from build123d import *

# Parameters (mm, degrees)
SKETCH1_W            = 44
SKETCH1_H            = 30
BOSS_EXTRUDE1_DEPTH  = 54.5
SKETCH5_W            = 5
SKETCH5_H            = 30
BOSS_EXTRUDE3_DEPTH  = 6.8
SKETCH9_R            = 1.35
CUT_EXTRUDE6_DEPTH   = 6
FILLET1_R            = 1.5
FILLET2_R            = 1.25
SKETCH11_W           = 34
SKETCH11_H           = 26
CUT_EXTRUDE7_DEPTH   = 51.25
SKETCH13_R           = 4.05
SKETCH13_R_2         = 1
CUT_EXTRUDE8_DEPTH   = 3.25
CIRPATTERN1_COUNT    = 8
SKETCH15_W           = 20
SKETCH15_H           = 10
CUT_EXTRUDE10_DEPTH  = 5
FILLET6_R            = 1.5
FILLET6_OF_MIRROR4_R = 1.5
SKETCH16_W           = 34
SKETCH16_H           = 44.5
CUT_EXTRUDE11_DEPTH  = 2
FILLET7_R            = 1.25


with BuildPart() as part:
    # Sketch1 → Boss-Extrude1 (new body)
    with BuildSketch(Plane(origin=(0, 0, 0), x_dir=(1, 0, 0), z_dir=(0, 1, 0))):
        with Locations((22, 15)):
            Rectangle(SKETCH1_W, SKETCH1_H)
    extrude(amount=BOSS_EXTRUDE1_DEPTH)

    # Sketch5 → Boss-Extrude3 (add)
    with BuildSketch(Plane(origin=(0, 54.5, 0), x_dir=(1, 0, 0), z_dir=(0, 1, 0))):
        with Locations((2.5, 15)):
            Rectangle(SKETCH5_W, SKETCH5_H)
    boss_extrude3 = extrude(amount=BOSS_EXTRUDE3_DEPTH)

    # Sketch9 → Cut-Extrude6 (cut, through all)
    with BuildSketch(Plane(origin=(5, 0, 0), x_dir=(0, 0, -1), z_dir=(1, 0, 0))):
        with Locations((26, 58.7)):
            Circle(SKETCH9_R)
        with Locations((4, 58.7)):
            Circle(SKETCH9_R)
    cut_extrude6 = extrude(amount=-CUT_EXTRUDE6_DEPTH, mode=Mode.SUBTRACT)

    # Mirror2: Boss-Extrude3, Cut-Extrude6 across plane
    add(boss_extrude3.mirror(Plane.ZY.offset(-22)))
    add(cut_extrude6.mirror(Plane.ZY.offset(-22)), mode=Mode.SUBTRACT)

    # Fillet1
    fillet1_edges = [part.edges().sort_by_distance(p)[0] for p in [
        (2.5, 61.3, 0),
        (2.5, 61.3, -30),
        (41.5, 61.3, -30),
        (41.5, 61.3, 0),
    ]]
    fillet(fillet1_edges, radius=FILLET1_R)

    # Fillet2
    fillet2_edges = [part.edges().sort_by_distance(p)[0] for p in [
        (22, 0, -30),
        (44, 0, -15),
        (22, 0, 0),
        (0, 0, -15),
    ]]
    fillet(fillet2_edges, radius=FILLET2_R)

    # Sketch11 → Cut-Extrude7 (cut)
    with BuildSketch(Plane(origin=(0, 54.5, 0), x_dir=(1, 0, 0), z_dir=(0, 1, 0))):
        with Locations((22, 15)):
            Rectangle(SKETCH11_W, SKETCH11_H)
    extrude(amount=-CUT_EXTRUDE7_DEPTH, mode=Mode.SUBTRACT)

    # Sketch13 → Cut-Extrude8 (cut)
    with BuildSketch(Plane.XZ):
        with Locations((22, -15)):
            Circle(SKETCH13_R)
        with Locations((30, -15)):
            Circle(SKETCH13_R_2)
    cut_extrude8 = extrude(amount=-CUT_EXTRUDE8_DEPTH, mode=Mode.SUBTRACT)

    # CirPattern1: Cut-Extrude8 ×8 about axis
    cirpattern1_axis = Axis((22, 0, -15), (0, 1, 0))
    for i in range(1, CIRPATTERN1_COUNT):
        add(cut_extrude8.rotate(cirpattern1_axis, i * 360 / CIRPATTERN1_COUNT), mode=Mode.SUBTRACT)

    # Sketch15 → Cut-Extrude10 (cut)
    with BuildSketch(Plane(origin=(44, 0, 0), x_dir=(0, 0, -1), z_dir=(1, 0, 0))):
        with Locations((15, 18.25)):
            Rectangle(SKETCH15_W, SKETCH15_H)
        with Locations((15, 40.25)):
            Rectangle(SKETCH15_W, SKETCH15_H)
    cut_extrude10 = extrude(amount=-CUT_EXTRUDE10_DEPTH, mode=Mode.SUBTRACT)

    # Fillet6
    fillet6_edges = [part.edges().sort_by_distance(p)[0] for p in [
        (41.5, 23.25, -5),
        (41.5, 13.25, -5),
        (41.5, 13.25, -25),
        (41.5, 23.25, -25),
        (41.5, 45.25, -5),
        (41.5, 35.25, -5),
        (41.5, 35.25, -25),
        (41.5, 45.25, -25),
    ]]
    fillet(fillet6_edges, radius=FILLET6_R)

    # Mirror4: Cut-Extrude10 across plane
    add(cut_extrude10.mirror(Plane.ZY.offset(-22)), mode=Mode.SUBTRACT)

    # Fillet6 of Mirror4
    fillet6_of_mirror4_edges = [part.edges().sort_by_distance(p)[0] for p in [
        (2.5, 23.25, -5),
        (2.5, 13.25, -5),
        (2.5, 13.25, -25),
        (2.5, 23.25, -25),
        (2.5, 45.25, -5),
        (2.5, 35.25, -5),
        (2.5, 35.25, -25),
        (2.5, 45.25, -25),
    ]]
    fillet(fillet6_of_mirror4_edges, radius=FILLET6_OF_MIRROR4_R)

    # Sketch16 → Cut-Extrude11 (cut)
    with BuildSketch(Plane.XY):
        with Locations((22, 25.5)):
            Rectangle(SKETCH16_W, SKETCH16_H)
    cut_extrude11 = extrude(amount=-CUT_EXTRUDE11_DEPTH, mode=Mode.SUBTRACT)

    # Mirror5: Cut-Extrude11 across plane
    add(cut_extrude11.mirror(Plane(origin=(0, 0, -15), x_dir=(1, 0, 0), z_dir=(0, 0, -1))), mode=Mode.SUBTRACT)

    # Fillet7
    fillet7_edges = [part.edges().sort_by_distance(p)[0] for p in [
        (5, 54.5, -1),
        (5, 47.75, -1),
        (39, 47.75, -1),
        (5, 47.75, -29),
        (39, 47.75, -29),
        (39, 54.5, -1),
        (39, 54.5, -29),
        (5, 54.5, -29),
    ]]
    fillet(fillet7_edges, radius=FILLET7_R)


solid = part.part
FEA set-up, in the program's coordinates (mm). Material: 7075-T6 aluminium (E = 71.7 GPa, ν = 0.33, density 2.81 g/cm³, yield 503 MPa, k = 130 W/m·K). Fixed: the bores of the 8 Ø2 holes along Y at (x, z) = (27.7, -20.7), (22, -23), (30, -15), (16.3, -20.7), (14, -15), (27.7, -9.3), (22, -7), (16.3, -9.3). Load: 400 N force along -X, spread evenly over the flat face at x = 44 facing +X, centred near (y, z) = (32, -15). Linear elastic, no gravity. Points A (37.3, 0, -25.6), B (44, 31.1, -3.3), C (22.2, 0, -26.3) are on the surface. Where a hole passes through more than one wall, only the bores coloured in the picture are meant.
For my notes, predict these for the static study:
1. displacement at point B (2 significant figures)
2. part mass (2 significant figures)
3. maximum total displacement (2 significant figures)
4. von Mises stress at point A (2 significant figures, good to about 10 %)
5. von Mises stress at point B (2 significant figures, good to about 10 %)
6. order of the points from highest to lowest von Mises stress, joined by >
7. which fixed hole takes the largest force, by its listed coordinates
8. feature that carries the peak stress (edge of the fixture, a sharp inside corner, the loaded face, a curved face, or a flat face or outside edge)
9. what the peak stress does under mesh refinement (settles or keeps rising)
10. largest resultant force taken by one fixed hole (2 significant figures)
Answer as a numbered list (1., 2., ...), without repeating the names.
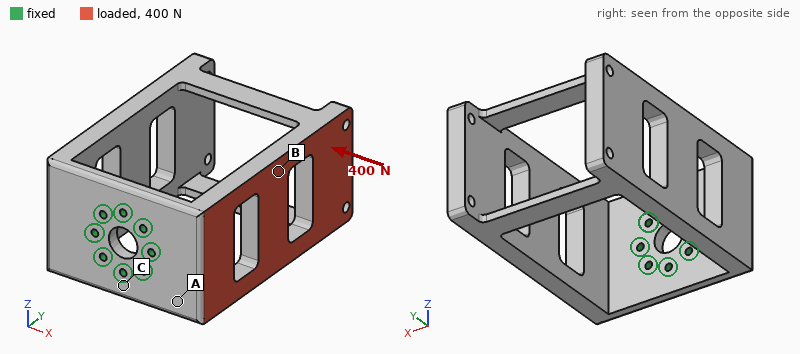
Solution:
1. 0.30 mm
2. 51 g
3. 0.48 mm
4. 68 MPa
5. 22 MPa
6. A > B > C
7. (30, -15)
8. edge of the fixture
9. keeps rising
10. 340 N
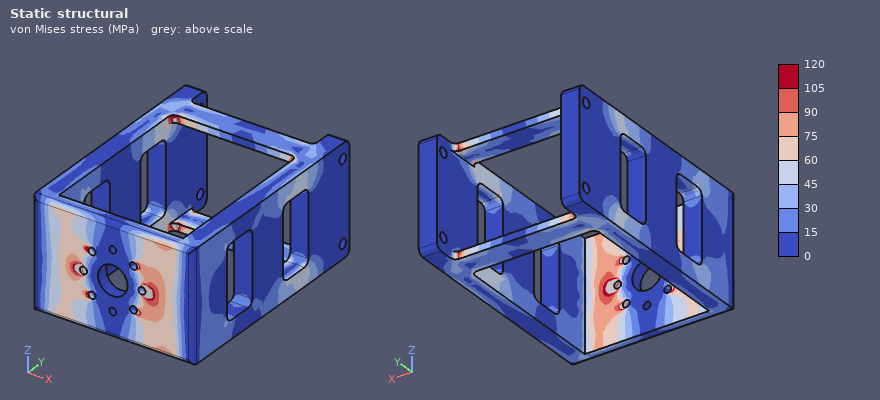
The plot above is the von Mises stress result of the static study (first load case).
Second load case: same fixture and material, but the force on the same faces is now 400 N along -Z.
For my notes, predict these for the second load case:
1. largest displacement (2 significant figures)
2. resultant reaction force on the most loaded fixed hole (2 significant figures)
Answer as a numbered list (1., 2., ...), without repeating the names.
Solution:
1. 0.37 mm
2. 530 N
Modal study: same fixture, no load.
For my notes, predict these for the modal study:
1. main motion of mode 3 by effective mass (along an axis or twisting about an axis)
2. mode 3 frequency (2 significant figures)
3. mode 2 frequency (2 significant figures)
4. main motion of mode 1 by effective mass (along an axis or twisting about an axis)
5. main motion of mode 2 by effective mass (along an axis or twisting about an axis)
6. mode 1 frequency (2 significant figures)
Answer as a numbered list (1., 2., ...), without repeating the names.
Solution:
1. twisting about Y
2. 1600 Hz
3. 1100 Hz
4. along X
5. along Z
6. 790 Hz
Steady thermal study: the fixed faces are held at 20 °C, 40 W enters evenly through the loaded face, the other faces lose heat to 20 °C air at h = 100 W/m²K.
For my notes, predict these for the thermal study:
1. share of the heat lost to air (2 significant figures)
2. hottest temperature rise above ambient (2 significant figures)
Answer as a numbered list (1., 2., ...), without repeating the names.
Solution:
1. 50 %
2. 60 K
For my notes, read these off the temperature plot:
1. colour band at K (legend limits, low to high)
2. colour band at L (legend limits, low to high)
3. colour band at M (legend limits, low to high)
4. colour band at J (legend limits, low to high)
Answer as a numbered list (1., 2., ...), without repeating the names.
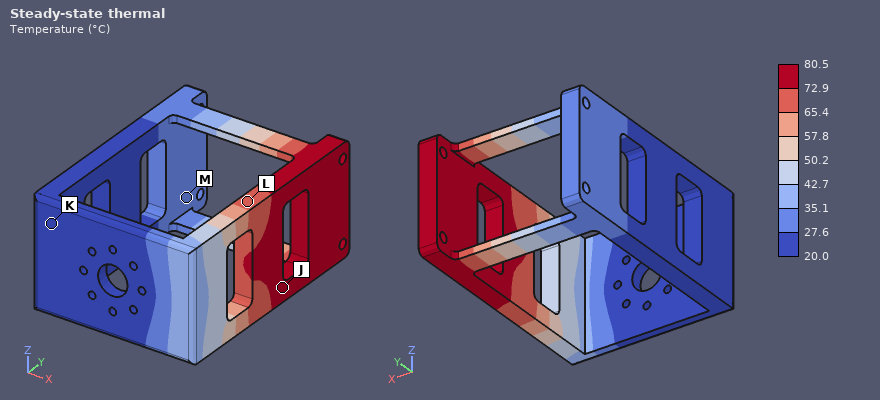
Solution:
1. 20.0 to 27.6 °C
2. 65.4 to 72.9 °C
3. 27.6 to 35.1 °C
4. 72.9 to 80.5 °C
